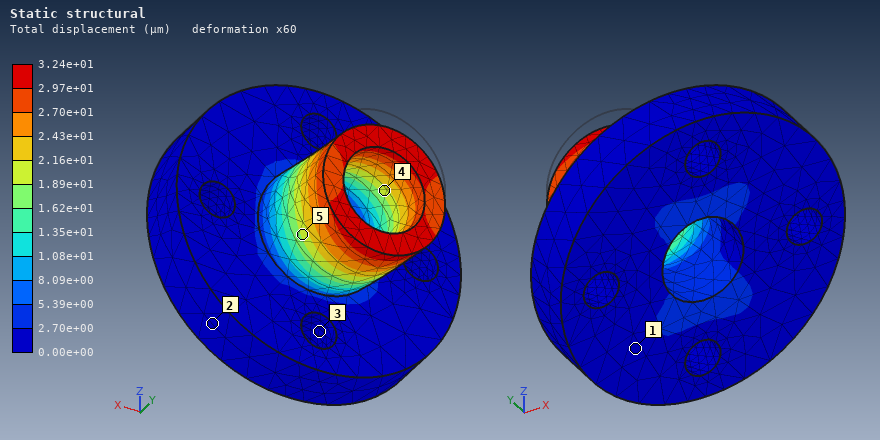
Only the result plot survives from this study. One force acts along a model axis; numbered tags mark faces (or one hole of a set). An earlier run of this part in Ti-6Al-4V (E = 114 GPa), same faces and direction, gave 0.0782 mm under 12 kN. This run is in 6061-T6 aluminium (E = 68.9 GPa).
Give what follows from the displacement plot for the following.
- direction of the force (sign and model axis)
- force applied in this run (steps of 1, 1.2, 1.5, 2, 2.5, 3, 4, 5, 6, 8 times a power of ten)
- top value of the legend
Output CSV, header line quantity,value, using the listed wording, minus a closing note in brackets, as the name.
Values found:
quantity,value
direction of the force,-Z
force applied in this run,3 kN
top value of the legend,3.24e+01 µm
